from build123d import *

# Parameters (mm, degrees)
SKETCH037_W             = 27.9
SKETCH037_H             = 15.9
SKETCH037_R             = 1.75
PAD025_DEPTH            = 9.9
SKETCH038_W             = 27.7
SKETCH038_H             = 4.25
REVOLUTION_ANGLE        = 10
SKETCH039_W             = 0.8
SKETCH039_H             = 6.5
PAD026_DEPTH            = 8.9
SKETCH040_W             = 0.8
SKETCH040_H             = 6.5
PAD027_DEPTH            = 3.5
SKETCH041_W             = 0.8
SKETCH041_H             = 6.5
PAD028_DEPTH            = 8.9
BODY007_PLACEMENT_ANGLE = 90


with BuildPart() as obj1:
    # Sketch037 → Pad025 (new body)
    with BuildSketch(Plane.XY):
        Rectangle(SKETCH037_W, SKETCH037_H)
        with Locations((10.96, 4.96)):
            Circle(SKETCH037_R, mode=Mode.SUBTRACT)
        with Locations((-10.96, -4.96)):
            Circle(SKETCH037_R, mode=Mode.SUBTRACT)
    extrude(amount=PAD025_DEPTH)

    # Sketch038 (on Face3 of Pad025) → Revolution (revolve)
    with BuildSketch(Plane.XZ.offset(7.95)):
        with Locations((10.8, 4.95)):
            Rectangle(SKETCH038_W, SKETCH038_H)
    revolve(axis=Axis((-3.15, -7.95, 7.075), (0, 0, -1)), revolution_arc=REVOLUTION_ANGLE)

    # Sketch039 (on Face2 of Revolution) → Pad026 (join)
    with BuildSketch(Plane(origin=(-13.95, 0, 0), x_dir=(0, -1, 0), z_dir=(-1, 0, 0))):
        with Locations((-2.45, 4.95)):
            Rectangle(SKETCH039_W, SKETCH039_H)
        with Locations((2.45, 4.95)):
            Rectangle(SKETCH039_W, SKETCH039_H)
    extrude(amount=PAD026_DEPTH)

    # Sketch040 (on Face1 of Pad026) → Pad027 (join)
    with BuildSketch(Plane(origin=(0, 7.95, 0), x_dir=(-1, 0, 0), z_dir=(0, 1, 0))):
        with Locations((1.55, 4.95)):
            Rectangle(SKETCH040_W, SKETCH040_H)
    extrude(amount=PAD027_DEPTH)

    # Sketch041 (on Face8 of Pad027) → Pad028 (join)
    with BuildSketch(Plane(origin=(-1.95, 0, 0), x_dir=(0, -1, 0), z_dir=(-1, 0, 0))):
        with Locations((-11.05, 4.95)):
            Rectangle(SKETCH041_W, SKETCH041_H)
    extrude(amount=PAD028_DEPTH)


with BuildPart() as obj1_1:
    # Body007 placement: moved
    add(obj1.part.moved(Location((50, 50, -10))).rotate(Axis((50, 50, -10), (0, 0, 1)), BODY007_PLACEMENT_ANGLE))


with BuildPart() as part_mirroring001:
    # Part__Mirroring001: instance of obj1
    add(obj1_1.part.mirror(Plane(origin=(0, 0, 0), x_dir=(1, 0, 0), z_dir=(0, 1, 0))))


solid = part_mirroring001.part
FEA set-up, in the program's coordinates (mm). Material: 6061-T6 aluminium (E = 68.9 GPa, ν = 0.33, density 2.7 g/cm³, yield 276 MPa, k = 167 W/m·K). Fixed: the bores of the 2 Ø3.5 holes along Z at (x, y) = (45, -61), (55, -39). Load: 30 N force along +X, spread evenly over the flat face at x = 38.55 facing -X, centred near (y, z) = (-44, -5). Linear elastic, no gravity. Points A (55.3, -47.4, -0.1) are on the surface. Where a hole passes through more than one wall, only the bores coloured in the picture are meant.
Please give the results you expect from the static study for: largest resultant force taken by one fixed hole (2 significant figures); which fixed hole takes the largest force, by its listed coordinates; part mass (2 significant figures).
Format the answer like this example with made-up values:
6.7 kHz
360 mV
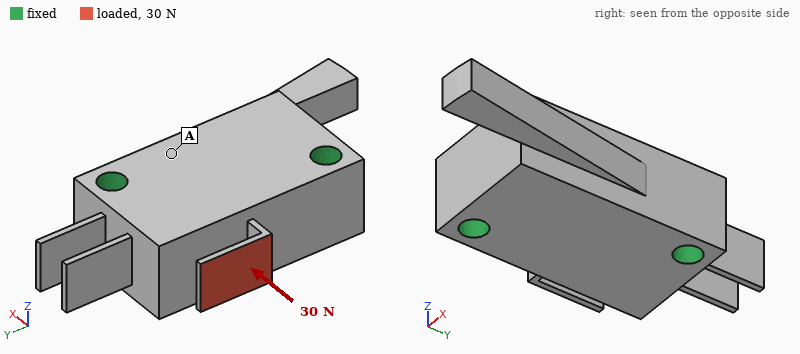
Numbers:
24 N
(55, -39)
13 g
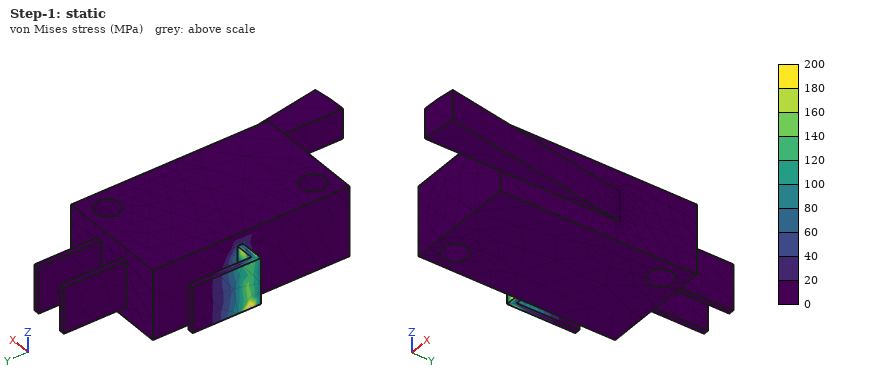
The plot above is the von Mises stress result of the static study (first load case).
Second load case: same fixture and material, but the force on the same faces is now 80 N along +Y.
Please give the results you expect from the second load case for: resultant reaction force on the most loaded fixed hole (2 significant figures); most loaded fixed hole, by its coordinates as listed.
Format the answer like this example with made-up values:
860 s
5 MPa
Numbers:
63 N
(45, -61)
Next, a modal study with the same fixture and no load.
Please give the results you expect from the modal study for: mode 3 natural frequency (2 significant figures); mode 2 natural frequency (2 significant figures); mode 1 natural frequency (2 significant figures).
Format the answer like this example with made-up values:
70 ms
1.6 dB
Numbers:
8100 Hz
8100 Hz
5100 Hz
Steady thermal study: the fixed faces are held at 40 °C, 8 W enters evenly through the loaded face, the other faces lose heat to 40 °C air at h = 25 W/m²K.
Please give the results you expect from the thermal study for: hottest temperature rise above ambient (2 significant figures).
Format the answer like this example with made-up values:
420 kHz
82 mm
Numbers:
73 K
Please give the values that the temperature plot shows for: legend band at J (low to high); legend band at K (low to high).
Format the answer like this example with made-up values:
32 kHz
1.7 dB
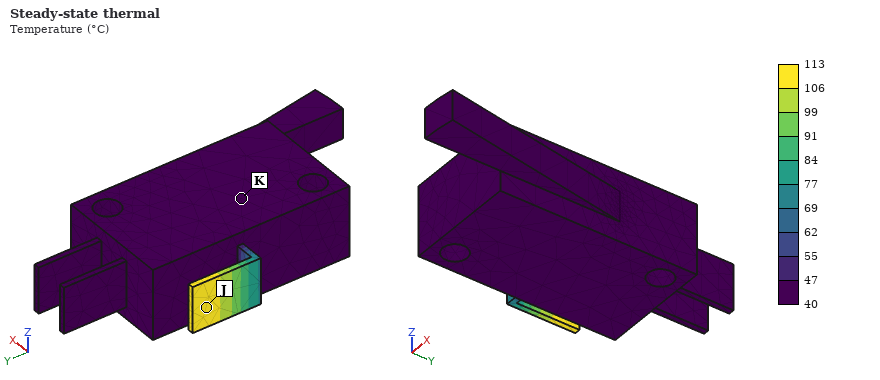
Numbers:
106 to 113 °C
40 to 47 °C
